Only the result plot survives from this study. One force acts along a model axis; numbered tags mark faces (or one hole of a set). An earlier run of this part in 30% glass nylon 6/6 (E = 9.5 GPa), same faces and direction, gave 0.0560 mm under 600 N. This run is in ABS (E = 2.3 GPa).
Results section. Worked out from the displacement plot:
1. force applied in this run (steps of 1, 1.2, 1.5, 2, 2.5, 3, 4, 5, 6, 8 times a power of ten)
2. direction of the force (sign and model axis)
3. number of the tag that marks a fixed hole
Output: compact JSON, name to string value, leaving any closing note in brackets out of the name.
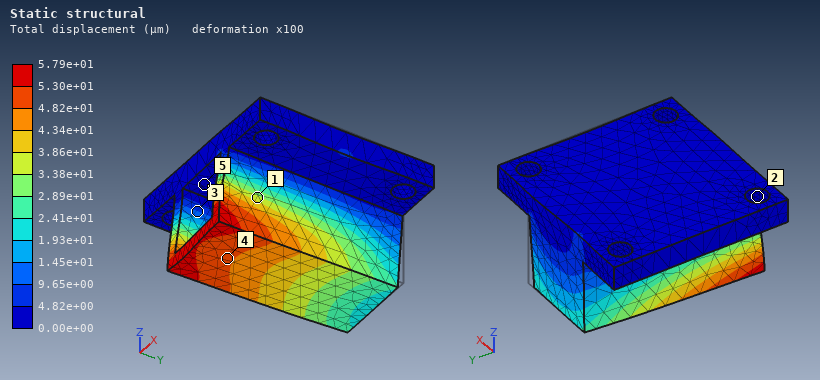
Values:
{"force applied in this run": "150 N", "direction of the force": "-X", "number of the tag that marks a fixed hole": "2"}
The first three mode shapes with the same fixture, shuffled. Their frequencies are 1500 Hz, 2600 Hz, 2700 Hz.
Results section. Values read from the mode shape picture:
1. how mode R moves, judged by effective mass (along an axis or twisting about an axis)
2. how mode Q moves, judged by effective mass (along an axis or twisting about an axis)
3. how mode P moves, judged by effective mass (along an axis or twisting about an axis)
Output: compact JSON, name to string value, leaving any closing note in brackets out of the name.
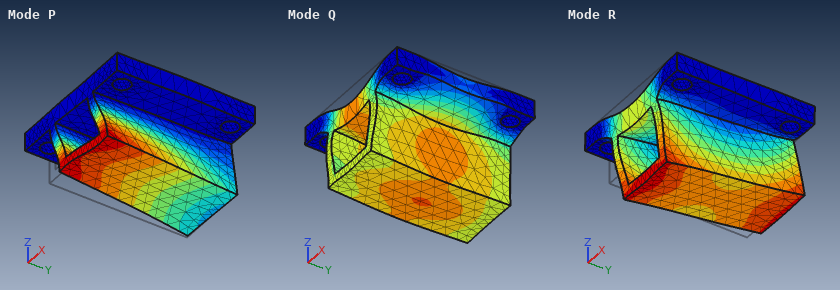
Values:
{"how mode R moves, judged by effective mass": "along Y", "how mode Q moves, judged by effective mass": "along Z", "how mode P moves, judged by effective mass": "along X"}
